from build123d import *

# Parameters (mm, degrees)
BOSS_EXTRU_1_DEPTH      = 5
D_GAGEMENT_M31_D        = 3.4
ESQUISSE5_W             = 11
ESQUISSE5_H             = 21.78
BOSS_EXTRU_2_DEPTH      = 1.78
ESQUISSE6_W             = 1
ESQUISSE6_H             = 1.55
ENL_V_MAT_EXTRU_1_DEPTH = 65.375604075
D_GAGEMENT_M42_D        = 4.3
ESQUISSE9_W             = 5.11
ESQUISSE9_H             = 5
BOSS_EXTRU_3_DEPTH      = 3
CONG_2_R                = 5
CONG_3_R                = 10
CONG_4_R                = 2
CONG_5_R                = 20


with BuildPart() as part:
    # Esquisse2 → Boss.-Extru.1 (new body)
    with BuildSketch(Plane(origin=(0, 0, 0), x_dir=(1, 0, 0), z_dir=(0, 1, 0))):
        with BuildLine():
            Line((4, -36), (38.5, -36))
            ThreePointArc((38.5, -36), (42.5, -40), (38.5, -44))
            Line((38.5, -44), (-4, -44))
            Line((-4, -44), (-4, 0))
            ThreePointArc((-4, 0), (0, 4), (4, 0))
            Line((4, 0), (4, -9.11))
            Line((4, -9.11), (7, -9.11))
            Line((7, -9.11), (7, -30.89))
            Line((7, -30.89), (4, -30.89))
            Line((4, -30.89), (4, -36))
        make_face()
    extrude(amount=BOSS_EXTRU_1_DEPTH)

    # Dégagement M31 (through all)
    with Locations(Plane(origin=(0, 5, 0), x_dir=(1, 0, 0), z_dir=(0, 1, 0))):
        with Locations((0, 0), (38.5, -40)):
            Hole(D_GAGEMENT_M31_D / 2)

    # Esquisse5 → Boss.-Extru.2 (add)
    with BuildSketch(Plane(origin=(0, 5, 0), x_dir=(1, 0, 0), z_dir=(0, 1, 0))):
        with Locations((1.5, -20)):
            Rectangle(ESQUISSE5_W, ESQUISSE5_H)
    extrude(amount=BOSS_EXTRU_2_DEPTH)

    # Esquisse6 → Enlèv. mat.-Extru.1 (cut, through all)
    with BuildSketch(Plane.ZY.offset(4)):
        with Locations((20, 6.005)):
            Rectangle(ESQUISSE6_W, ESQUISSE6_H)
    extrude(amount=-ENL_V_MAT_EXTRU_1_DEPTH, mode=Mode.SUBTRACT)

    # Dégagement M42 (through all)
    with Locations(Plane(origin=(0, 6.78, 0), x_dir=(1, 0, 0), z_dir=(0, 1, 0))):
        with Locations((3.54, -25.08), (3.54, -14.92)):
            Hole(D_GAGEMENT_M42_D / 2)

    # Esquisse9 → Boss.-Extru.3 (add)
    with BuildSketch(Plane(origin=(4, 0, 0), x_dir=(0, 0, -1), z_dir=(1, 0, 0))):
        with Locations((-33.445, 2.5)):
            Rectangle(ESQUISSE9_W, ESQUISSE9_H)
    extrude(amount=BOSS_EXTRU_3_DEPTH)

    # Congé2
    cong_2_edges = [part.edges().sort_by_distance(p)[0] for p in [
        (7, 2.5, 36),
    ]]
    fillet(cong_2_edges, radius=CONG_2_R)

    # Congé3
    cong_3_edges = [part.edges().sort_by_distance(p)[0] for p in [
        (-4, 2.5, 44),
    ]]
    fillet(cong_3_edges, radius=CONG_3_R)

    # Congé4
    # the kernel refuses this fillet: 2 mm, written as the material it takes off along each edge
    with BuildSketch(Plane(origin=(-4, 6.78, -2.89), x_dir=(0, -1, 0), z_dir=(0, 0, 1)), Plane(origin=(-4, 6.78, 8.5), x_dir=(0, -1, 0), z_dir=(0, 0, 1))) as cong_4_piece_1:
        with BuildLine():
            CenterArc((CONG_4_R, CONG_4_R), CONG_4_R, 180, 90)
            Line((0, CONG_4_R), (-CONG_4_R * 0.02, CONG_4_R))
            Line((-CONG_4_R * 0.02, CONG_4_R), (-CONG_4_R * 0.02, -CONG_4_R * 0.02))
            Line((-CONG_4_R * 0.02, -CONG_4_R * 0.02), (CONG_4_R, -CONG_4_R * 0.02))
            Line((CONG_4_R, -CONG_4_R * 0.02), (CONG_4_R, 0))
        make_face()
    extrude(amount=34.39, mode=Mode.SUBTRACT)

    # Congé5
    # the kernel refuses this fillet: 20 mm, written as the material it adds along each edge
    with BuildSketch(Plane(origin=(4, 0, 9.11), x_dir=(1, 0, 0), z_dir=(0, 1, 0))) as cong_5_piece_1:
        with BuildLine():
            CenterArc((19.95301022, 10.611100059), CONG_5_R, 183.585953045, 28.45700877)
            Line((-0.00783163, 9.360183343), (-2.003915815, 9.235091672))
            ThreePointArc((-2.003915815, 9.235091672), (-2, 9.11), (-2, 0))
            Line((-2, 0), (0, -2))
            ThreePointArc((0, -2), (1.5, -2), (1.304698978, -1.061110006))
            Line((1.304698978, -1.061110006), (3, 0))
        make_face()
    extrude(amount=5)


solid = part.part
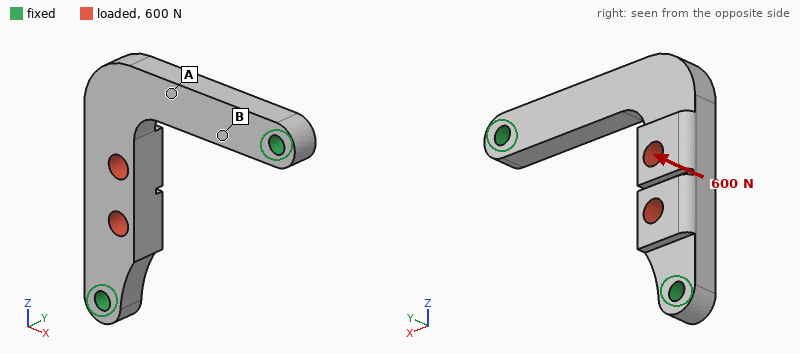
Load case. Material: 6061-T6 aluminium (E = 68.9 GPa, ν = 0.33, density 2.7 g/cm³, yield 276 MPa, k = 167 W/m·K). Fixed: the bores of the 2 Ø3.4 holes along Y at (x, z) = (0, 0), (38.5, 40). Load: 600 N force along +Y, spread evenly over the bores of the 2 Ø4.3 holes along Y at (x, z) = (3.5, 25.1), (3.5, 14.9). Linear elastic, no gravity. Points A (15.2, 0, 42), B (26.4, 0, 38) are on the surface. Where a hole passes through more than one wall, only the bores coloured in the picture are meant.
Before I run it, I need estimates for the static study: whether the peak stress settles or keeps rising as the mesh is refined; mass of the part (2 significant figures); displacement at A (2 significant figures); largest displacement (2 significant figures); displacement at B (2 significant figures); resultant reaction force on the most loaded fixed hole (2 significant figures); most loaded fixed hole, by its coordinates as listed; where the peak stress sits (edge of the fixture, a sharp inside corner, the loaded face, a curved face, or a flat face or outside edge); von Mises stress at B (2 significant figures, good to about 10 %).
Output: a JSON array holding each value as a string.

["keeps rising", "10 g", "0.094 mm", "0.18 mm", "0.030 mm", "460 N", "(0, 0)", "edge of the fixture", "44 MPa"]
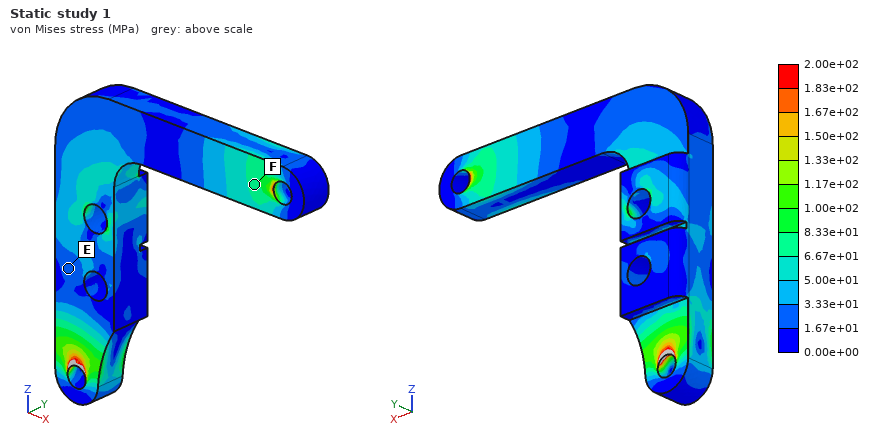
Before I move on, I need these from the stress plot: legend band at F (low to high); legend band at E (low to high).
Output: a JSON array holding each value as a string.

["6.67e+01 to 8.33e+01 MPa", "1.67e+01 to 3.33e+01 MPa"]
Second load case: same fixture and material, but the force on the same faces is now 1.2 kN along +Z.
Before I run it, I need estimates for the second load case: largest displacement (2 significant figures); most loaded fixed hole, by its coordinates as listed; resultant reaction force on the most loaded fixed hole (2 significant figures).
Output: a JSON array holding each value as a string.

["25 µm", "(0, 0)", "1.2 kN"]
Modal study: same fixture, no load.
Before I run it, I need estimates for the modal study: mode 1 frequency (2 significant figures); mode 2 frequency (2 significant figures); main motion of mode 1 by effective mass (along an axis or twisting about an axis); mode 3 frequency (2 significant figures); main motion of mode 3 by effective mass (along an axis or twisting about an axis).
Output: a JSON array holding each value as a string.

["3400 Hz", "12 kHz", "along Y", "15 kHz", "along X"]
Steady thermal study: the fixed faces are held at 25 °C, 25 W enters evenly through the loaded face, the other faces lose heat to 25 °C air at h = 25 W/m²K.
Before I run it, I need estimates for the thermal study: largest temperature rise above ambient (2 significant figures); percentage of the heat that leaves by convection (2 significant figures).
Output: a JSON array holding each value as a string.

["39 K", "5.0 %"]
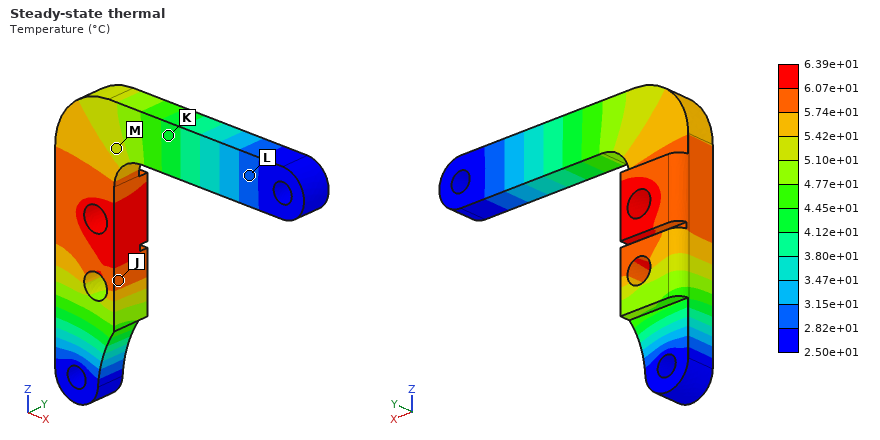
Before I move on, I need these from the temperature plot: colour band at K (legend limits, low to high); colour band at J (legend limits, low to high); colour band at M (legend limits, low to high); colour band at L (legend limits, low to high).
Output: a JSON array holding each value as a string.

["4.12e+01 to 4.45e+01 °C", "5.74e+01 to 6.07e+01 °C", "5.10e+01 to 5.42e+01 °C", "2.82e+01 to 3.15e+01 °C"]
